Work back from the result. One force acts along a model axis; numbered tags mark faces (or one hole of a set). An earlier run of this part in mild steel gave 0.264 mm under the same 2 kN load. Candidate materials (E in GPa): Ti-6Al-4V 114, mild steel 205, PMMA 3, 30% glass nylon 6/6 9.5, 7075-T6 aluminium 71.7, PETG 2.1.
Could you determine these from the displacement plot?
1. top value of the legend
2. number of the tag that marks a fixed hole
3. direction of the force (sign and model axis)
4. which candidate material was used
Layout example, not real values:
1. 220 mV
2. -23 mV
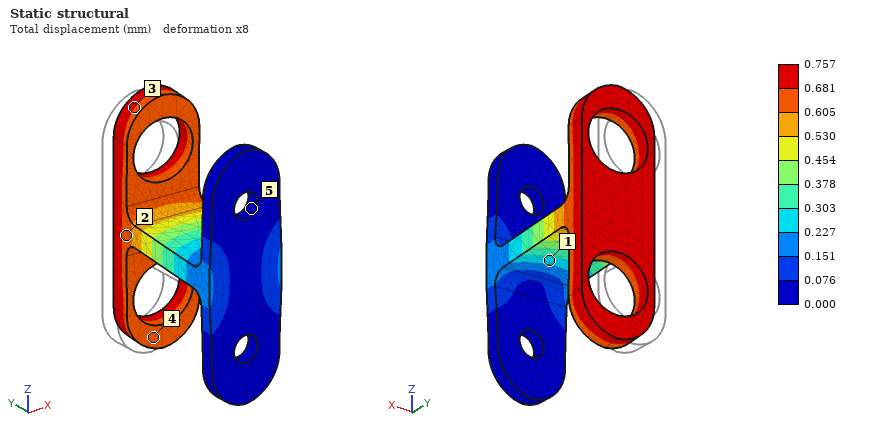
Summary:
1. 0.757 mm
2. 5
3. +X
4. 7075-T6 aluminium
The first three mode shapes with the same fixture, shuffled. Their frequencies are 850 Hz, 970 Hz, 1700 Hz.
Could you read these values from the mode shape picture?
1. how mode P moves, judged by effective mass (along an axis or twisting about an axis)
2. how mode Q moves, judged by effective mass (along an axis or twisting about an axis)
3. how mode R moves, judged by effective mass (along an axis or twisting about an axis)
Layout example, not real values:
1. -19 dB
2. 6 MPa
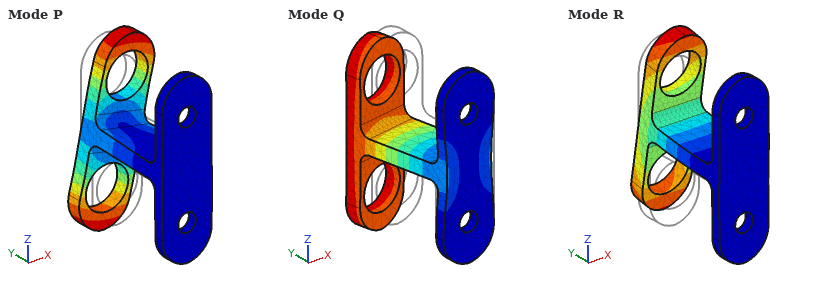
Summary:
1. twisting about Y
2. along X
3. along Z
